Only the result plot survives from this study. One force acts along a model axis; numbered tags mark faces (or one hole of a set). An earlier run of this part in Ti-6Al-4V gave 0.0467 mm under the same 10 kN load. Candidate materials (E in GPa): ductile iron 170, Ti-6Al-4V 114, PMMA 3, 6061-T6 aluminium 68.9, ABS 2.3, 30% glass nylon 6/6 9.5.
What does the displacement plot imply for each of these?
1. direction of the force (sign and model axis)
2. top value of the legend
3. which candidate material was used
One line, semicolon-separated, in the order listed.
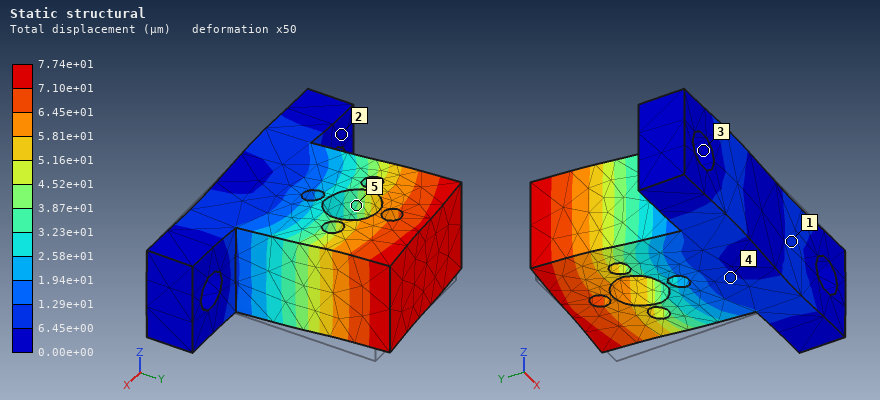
-X; 7.74e+01 µm; 6061-T6 aluminium
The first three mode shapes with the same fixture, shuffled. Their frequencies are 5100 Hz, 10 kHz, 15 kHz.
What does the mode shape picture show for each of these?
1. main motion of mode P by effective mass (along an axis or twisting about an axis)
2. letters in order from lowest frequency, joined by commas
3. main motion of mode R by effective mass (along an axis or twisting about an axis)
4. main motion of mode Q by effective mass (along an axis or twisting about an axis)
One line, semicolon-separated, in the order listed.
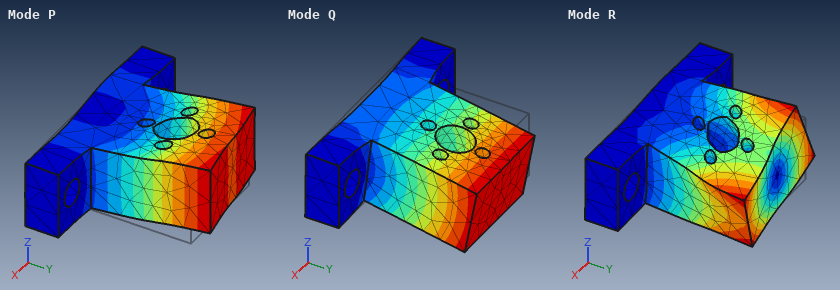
along X; Q, P, R; twisting about Y; along Z
